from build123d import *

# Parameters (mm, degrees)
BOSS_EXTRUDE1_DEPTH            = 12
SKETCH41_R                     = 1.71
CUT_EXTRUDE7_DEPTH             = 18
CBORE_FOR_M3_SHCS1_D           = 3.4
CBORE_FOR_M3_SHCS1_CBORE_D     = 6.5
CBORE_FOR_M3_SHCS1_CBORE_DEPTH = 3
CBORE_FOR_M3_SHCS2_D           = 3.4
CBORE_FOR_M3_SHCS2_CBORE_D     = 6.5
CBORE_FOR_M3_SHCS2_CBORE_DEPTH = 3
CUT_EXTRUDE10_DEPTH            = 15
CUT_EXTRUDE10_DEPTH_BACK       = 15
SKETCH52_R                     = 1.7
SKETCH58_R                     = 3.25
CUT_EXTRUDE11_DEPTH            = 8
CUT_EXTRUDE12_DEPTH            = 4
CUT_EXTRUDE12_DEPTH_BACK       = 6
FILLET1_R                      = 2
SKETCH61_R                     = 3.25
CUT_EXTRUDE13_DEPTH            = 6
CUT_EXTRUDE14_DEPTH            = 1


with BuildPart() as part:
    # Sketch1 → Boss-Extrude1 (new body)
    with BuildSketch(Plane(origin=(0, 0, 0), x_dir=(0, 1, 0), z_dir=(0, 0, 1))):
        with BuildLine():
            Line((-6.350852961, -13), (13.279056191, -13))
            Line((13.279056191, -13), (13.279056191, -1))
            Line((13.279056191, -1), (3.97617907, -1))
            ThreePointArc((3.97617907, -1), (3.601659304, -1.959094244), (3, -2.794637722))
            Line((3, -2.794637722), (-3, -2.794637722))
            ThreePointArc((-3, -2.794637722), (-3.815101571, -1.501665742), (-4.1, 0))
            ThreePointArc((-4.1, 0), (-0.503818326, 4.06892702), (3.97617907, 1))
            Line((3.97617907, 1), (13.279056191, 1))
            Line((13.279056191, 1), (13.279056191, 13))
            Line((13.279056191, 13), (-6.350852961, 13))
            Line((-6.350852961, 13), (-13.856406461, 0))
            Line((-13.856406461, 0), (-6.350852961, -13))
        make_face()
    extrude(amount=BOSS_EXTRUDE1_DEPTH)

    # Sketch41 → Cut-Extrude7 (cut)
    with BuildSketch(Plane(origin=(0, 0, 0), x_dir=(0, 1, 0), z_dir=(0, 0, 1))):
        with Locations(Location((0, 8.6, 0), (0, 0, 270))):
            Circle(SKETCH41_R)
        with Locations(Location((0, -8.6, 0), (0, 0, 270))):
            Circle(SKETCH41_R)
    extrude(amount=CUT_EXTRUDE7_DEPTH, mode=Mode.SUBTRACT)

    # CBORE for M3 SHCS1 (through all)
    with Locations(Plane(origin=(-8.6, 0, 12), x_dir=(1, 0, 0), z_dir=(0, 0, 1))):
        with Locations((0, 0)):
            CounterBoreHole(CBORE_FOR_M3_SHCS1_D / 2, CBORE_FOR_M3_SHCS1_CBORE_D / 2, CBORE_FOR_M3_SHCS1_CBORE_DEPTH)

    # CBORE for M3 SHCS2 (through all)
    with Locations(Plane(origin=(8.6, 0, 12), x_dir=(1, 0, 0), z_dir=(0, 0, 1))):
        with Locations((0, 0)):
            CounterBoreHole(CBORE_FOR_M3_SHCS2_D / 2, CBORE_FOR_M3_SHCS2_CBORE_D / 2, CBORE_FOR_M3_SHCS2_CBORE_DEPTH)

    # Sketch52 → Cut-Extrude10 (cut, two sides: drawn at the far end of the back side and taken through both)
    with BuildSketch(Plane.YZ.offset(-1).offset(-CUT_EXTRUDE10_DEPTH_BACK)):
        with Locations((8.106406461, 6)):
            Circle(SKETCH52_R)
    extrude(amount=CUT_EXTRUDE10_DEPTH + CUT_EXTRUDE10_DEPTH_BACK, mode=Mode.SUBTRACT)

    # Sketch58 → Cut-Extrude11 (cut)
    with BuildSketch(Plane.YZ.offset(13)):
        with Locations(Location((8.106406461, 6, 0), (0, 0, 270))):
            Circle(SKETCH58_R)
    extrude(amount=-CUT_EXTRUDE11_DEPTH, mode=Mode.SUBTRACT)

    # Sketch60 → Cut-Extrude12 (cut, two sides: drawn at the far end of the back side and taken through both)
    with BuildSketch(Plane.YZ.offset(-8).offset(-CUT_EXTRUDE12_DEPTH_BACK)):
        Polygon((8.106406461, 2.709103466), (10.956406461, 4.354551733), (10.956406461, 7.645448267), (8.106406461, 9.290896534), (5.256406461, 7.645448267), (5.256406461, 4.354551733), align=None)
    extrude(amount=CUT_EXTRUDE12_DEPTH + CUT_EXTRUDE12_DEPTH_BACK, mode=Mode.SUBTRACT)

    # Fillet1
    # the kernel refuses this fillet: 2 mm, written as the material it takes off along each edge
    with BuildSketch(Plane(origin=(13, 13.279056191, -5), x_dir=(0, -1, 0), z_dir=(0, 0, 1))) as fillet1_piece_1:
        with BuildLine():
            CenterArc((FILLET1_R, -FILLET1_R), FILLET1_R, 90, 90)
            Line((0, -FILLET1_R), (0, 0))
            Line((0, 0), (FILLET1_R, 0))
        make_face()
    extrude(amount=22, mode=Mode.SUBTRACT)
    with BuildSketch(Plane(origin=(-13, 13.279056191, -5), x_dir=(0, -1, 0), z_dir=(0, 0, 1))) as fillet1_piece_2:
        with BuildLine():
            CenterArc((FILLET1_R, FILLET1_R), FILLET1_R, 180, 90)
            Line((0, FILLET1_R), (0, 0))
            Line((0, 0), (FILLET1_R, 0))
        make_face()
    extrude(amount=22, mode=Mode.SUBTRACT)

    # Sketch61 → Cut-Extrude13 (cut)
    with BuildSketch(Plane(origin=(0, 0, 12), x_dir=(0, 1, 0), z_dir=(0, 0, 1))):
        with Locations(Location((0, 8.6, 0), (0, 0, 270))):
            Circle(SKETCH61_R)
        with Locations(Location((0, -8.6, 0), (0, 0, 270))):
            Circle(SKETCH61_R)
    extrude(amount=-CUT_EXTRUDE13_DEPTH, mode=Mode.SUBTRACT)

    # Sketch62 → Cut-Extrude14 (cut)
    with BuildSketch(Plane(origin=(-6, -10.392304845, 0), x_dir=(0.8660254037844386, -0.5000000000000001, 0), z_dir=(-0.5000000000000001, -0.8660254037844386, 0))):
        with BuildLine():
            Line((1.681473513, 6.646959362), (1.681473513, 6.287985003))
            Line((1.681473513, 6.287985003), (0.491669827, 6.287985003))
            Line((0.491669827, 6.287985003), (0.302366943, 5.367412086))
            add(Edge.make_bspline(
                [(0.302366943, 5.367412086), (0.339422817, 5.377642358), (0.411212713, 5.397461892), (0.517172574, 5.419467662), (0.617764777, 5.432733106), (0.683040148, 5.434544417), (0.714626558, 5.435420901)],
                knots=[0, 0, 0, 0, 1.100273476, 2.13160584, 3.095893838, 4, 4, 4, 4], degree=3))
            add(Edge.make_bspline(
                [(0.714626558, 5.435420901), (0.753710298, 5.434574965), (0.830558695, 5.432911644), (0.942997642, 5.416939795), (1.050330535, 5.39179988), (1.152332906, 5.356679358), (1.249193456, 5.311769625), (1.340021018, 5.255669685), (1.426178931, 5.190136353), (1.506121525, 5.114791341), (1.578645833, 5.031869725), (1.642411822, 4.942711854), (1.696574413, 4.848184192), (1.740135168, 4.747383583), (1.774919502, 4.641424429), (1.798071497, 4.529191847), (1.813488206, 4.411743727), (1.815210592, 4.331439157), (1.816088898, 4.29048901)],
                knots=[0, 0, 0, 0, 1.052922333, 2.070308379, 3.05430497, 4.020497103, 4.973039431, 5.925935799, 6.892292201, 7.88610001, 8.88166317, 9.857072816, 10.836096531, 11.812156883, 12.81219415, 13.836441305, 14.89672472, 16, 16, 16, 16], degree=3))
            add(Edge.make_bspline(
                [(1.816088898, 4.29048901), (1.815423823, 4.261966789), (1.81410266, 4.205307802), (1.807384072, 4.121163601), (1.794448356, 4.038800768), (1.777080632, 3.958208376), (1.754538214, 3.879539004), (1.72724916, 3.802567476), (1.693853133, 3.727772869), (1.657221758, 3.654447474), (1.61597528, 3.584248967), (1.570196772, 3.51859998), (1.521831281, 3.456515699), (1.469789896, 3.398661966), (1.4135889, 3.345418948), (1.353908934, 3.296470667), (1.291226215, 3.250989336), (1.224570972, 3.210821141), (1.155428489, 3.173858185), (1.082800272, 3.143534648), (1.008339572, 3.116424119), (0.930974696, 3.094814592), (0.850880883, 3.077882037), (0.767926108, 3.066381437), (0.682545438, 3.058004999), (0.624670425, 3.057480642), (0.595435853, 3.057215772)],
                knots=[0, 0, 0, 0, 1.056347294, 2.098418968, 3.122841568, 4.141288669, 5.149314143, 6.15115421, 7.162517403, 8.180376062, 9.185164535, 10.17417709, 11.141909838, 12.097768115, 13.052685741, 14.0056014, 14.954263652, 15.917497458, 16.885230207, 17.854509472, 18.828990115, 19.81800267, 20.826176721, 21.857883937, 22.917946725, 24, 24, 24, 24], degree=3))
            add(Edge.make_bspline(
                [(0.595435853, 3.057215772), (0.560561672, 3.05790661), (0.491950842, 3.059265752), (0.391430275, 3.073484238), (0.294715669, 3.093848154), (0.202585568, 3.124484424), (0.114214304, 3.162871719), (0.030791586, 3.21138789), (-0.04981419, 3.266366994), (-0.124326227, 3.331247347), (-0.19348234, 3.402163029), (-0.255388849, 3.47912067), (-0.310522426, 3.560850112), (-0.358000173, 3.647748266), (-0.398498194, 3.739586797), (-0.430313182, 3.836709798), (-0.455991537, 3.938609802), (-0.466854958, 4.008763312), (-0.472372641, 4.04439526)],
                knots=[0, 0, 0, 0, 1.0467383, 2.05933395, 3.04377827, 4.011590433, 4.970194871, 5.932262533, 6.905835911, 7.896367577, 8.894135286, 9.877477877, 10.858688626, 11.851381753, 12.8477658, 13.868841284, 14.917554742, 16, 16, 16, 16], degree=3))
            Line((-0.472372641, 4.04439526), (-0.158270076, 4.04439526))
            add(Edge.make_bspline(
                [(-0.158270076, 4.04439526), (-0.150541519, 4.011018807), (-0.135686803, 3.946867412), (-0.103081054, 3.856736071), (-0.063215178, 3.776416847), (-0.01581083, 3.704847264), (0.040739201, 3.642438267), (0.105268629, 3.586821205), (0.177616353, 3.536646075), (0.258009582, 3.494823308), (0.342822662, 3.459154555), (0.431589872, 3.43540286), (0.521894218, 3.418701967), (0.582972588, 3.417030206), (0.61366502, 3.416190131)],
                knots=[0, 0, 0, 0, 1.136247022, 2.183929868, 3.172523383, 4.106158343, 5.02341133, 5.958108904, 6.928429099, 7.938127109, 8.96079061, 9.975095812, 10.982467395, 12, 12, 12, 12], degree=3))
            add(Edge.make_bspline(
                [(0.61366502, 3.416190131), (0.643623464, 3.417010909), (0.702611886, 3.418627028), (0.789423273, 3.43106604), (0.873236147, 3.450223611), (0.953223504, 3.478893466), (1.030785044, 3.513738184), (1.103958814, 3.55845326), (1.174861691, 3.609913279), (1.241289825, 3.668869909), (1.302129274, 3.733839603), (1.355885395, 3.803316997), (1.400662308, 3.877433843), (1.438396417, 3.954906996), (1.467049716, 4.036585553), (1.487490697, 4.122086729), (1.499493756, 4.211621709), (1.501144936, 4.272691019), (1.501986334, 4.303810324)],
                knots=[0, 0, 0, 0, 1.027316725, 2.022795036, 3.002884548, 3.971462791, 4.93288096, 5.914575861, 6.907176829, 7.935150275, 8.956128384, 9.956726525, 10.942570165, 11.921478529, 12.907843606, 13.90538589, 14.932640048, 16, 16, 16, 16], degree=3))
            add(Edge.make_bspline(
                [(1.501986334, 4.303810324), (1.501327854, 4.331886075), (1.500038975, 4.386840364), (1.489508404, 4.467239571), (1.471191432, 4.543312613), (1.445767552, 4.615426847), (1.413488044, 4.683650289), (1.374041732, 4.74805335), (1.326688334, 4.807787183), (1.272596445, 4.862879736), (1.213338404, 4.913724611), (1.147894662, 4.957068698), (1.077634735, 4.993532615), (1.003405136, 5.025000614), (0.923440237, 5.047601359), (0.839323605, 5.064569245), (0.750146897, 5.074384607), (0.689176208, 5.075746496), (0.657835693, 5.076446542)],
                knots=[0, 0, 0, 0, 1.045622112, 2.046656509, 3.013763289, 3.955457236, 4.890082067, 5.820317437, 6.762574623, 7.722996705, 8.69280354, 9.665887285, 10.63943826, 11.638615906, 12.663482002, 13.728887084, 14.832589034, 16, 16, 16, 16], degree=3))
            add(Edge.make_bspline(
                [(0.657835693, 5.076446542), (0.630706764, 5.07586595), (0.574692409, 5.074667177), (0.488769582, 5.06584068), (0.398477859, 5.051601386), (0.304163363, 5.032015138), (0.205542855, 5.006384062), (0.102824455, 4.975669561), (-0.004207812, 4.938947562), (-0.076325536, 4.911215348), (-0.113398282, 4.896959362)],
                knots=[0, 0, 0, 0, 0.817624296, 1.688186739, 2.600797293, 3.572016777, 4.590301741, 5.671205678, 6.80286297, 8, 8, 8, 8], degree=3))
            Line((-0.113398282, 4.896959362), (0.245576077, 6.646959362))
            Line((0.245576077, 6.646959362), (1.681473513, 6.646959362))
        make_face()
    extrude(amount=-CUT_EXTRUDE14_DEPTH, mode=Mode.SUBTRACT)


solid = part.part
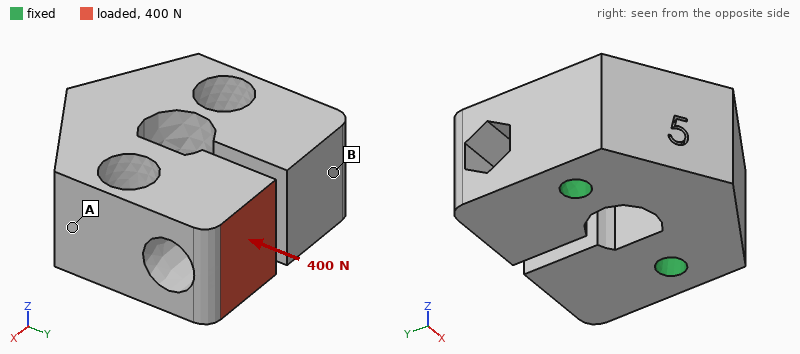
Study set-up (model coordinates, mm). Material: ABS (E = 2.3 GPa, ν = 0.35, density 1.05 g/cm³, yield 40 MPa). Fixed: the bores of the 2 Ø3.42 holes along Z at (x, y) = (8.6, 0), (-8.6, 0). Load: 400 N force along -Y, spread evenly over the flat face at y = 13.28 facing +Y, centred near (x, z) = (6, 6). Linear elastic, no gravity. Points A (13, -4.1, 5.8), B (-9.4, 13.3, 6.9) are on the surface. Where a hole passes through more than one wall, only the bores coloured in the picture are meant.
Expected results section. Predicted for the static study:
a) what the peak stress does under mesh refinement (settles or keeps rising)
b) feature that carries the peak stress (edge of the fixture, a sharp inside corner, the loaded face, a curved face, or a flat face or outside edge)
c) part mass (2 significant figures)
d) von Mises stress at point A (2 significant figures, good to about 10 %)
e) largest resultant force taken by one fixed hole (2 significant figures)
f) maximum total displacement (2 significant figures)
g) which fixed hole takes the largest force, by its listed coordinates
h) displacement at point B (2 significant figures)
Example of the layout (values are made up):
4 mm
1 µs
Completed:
keeps rising
edge of the fixture
5.7 g
2.8 MPa
360 N
0.12 mm
(8.6, 0)
0.021 mm
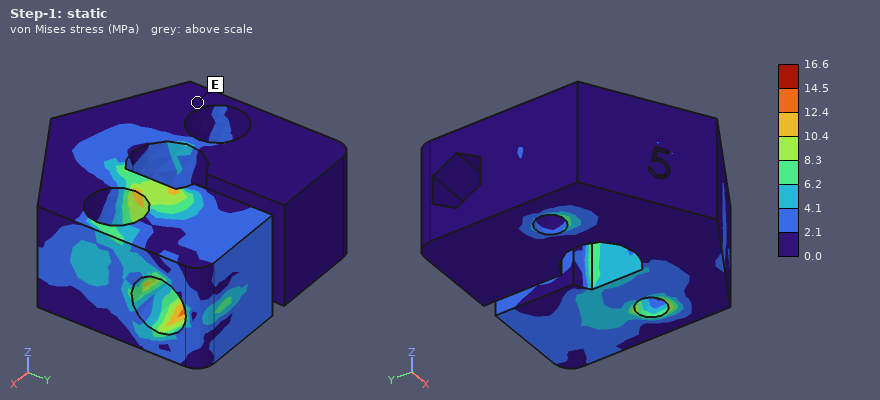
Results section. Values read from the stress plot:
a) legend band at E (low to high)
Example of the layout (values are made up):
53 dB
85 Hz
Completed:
0.0 to 2.1 MPa
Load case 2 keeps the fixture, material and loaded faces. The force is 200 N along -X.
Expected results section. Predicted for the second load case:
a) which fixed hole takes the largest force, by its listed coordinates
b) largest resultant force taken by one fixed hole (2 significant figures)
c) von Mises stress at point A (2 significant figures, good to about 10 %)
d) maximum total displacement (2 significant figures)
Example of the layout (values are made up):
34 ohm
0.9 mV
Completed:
(8.6, 0)
280 N
5.0 MPa
0.25 mm
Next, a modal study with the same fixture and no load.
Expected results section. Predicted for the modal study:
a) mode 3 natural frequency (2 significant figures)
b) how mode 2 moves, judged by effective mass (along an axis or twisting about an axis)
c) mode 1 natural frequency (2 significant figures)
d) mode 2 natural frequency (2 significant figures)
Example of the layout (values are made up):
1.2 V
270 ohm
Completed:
6000 Hz
along X
5000 Hz
5700 Hz
